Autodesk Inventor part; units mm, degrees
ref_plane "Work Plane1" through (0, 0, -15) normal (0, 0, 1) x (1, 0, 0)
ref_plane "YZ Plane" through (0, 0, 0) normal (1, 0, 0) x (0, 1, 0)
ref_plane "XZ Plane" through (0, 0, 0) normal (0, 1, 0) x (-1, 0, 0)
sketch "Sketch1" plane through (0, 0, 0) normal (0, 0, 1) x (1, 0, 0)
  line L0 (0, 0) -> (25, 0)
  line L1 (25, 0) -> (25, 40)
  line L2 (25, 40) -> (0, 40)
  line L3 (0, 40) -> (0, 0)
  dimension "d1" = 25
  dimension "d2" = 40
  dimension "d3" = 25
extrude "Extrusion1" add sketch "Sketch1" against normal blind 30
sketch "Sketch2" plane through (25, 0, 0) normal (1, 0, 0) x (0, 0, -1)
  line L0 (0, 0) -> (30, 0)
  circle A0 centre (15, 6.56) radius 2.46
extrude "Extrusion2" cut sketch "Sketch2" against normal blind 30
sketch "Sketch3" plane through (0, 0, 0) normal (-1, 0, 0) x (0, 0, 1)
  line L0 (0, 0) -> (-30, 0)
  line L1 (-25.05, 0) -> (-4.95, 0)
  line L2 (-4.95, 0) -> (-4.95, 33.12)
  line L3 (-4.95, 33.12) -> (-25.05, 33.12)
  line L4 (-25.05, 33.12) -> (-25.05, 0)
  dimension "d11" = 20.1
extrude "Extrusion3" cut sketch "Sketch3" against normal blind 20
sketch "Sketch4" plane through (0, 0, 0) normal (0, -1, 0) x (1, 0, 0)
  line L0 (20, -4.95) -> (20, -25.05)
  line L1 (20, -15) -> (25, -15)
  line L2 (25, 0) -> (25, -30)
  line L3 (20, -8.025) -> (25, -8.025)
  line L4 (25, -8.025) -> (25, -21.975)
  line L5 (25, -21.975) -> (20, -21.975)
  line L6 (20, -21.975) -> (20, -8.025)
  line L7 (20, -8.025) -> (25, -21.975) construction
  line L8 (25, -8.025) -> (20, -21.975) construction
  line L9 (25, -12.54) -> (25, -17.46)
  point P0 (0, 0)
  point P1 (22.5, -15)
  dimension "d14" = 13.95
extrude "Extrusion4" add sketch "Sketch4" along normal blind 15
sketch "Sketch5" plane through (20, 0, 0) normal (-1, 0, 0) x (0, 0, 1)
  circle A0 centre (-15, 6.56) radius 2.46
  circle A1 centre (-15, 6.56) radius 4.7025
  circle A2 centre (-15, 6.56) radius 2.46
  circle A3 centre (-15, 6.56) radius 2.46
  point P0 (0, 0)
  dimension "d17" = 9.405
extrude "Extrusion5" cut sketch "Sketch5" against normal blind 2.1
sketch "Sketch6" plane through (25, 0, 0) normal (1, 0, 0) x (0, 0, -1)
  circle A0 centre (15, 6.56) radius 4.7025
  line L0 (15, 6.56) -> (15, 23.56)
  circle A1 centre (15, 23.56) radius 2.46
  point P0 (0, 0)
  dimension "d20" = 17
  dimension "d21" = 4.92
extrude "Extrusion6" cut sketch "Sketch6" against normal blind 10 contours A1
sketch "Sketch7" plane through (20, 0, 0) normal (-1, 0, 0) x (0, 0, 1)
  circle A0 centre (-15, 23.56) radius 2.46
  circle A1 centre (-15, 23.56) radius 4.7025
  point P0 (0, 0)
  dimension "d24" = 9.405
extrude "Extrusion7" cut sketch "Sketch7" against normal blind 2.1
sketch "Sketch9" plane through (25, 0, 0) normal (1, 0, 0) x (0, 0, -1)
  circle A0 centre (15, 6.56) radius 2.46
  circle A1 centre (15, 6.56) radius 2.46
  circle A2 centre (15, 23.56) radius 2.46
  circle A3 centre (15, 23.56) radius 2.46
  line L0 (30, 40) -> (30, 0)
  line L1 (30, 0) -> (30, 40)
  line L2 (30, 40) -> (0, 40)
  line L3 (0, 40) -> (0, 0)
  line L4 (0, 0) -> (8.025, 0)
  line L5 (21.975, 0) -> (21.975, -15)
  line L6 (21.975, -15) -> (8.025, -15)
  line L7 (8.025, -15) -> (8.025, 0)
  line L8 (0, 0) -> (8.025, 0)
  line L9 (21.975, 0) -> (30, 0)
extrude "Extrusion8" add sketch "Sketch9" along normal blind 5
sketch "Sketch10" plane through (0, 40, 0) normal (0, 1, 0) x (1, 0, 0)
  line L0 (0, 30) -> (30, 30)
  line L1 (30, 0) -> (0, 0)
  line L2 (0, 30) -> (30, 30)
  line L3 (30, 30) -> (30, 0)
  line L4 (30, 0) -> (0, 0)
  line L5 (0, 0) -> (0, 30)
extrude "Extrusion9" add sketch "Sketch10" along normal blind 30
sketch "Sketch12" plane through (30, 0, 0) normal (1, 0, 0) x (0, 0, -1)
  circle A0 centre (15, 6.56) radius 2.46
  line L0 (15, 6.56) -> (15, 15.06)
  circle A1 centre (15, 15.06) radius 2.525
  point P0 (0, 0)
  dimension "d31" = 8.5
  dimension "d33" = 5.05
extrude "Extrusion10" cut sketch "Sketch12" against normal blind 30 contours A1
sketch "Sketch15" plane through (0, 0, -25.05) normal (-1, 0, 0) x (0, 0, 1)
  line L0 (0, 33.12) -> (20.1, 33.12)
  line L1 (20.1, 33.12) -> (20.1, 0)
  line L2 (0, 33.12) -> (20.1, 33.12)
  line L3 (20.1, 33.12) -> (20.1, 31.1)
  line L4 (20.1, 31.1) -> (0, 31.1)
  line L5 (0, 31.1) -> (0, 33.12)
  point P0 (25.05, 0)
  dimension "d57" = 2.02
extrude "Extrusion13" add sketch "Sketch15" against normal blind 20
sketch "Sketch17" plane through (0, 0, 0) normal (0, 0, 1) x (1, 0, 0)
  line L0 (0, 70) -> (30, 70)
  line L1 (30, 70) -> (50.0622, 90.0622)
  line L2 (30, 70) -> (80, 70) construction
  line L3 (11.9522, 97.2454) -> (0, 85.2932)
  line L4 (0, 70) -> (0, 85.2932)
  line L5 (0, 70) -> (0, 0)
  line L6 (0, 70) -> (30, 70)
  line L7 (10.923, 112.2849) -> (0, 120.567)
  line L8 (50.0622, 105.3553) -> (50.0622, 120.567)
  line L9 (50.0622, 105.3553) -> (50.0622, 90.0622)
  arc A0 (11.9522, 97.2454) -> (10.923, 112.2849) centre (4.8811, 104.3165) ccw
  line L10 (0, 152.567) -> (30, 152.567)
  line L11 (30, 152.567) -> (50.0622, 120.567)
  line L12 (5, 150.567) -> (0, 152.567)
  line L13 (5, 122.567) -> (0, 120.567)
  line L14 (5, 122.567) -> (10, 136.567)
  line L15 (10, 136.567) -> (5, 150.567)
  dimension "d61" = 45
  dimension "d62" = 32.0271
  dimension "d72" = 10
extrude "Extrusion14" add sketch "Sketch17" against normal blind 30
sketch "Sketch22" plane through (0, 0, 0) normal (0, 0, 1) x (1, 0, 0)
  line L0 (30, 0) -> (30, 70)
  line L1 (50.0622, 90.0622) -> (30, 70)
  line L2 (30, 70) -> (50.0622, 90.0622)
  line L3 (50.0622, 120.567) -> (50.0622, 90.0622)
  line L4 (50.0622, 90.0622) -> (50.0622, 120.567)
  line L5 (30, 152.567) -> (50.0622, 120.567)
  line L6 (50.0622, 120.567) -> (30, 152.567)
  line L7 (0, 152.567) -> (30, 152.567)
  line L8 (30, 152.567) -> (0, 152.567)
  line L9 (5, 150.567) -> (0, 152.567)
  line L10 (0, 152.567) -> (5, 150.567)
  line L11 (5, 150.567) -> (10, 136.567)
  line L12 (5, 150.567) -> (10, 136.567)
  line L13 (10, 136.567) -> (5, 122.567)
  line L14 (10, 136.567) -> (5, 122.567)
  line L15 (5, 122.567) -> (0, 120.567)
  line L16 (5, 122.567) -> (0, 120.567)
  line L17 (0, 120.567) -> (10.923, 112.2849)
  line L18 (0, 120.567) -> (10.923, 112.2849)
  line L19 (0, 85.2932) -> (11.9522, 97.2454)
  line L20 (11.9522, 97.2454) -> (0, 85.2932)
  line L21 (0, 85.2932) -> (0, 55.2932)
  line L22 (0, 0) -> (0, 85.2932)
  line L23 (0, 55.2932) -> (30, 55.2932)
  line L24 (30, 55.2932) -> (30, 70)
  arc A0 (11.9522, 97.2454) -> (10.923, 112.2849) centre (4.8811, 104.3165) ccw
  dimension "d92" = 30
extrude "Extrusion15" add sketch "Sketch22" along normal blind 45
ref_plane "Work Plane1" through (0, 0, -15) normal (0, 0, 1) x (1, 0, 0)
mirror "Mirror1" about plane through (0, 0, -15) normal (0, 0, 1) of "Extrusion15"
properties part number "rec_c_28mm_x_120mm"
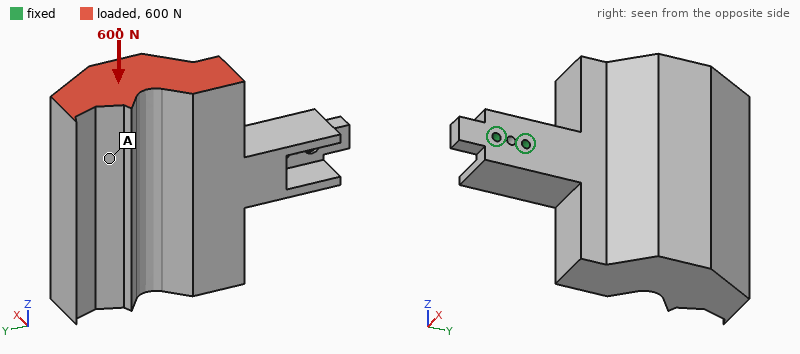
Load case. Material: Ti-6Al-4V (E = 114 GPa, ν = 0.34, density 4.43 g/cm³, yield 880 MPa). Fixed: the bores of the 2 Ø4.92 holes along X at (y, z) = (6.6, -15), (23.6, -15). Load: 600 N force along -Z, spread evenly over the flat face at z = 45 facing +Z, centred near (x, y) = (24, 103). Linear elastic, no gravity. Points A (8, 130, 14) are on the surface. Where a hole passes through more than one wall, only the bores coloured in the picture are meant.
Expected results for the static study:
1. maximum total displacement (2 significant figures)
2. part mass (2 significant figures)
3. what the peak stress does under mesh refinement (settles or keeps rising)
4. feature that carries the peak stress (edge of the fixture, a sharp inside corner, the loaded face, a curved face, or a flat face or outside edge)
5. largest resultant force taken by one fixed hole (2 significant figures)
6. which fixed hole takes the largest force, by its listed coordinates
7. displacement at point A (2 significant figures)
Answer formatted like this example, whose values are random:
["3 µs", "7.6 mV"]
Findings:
["86 µm", "2.0 kg", "keeps rising", "edge of the fixture", "2.7 kN", "(23.6, -15)", "62 µm"]
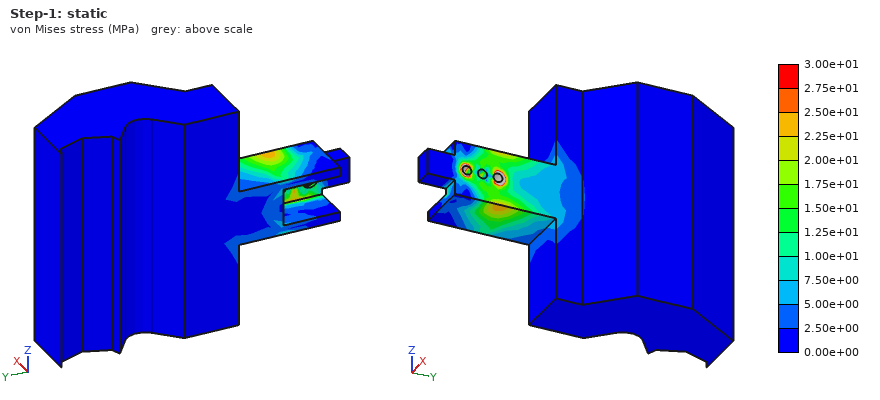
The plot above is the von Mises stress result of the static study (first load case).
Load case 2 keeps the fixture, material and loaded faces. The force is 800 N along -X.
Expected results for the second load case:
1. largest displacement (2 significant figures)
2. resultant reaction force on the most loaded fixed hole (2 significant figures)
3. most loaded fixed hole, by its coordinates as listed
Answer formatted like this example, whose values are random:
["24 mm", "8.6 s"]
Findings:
["0.24 mm", "3.3 kN", "(23.6, -15)"]
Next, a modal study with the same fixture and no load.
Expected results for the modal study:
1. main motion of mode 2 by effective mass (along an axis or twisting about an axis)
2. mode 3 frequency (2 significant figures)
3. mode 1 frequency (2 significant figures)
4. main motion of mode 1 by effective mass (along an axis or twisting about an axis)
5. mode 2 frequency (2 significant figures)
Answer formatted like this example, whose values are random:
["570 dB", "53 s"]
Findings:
["along Z", "550 Hz", "340 Hz", "along X", "360 Hz"]
